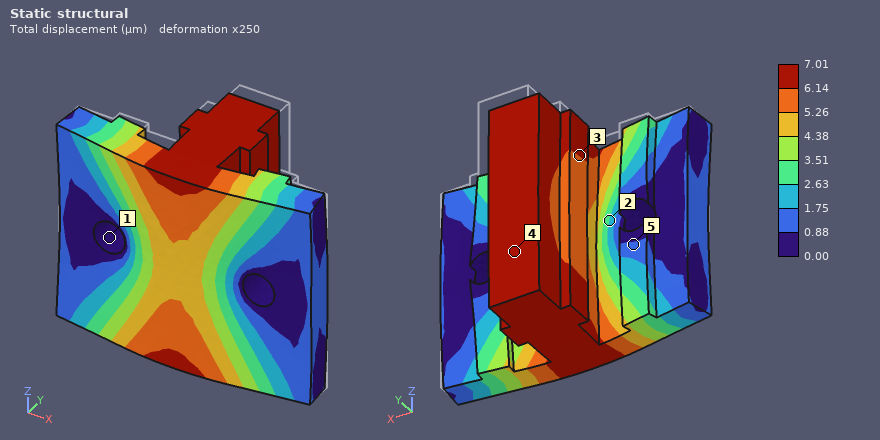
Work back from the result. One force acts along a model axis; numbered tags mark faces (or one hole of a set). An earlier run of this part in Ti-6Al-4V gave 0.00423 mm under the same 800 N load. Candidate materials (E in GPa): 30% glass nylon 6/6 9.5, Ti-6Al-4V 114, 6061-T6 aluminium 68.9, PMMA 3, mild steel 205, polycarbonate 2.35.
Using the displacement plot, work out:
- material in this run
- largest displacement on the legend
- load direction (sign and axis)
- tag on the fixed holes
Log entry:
6061-T6 aluminium
7.01 µm
-Y
1
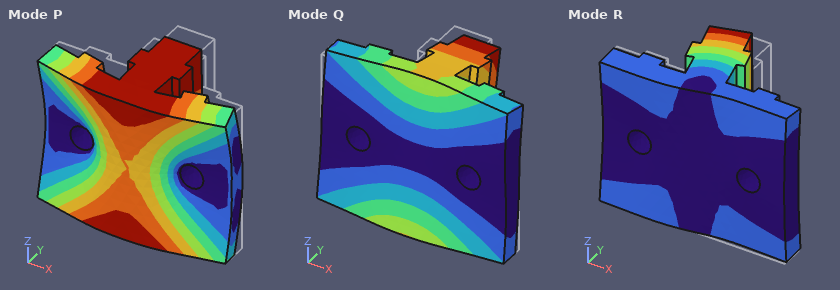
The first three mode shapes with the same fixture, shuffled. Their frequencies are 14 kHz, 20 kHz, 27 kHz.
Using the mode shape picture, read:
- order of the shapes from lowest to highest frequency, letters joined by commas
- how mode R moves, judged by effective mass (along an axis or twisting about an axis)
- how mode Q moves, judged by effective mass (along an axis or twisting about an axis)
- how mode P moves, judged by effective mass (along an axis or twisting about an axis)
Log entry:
Q, R, P
along X
along Z
along Y
